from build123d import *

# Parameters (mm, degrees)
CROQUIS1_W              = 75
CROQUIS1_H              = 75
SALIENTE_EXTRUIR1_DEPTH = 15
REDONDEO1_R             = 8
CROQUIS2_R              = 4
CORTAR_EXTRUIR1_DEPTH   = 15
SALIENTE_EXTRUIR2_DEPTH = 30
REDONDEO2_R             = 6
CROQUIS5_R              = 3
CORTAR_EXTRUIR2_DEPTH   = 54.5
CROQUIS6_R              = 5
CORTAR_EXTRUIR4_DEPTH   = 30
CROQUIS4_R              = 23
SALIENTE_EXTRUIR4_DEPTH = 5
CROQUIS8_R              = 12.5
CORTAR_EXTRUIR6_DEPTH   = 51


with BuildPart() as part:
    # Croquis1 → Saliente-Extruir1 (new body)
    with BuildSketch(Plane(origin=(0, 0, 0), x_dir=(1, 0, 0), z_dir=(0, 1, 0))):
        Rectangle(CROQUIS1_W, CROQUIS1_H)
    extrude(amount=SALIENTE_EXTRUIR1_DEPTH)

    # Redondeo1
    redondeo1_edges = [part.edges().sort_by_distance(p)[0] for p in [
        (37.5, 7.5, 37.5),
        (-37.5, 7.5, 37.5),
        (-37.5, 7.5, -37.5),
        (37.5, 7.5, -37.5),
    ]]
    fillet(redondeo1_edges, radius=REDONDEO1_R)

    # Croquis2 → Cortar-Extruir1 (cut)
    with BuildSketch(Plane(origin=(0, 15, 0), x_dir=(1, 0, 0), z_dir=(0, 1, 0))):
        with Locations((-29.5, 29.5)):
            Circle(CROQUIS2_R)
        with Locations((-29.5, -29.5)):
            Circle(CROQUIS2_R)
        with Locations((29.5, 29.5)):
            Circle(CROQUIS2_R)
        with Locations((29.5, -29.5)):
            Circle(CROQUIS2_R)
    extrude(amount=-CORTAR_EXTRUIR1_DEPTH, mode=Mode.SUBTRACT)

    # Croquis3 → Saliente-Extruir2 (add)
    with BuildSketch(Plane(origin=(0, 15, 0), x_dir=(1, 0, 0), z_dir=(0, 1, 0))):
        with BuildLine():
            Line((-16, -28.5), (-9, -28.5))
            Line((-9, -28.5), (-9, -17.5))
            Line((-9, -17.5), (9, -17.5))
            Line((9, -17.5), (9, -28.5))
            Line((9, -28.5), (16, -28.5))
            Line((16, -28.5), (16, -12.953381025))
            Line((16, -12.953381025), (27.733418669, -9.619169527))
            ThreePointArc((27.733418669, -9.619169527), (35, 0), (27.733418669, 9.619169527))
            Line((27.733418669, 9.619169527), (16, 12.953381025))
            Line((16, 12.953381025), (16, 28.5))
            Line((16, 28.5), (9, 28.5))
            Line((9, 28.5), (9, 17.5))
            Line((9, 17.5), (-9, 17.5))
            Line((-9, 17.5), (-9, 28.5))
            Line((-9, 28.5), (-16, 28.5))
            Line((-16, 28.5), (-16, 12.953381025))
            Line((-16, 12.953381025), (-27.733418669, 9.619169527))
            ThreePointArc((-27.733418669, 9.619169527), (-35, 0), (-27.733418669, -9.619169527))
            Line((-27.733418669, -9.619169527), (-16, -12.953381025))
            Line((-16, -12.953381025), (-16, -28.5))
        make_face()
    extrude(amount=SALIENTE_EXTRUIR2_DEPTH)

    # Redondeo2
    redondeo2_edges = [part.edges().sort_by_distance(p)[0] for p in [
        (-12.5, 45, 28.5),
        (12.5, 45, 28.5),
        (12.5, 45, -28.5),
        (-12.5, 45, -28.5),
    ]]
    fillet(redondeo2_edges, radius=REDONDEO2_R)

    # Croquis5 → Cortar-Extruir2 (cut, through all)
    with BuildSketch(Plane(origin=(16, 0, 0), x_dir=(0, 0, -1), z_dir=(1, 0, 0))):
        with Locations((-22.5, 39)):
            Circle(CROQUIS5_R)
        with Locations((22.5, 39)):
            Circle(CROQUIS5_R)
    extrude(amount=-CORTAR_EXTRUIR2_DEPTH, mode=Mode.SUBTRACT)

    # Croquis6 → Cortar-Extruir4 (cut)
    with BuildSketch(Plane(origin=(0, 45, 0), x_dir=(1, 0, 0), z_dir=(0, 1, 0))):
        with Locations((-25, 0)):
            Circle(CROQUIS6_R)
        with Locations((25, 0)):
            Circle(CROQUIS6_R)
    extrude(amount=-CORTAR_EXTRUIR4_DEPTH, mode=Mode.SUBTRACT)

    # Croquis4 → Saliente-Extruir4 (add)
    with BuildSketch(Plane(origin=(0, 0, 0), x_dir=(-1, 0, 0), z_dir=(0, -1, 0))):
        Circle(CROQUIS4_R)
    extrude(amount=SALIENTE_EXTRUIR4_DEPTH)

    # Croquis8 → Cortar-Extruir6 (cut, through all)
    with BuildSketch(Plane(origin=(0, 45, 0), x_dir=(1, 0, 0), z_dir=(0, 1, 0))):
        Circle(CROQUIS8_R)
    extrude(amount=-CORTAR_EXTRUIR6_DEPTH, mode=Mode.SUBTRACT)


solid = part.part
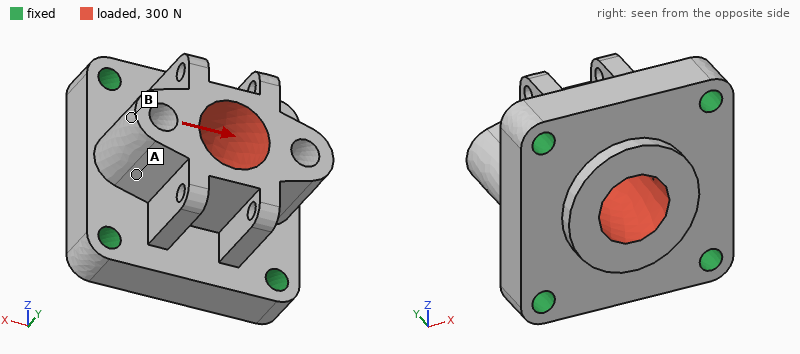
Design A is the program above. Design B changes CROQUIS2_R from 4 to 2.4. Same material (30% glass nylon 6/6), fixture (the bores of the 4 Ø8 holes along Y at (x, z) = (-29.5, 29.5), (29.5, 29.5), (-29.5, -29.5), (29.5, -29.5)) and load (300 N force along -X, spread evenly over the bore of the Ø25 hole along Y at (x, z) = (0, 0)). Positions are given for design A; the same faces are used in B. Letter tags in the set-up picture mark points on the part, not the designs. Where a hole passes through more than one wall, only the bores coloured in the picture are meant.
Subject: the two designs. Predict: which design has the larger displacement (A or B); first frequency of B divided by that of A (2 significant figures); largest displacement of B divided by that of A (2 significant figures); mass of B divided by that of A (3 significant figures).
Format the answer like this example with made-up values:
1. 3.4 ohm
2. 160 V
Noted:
1. B
2. 0.93
3. 1.1
4. 1.02
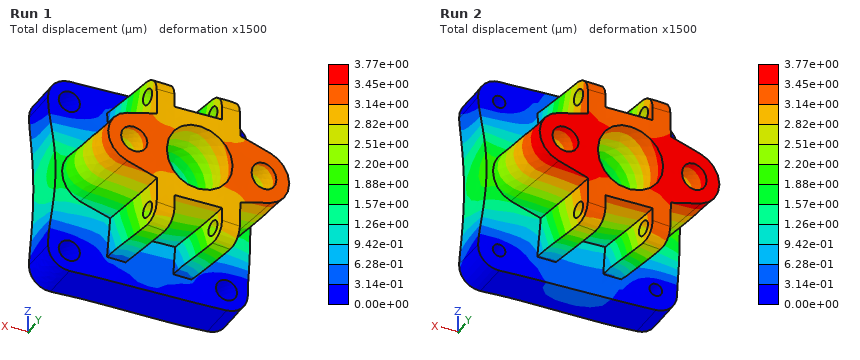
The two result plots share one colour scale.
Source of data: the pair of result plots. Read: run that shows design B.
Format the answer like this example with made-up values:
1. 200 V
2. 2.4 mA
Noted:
1. Run 2
